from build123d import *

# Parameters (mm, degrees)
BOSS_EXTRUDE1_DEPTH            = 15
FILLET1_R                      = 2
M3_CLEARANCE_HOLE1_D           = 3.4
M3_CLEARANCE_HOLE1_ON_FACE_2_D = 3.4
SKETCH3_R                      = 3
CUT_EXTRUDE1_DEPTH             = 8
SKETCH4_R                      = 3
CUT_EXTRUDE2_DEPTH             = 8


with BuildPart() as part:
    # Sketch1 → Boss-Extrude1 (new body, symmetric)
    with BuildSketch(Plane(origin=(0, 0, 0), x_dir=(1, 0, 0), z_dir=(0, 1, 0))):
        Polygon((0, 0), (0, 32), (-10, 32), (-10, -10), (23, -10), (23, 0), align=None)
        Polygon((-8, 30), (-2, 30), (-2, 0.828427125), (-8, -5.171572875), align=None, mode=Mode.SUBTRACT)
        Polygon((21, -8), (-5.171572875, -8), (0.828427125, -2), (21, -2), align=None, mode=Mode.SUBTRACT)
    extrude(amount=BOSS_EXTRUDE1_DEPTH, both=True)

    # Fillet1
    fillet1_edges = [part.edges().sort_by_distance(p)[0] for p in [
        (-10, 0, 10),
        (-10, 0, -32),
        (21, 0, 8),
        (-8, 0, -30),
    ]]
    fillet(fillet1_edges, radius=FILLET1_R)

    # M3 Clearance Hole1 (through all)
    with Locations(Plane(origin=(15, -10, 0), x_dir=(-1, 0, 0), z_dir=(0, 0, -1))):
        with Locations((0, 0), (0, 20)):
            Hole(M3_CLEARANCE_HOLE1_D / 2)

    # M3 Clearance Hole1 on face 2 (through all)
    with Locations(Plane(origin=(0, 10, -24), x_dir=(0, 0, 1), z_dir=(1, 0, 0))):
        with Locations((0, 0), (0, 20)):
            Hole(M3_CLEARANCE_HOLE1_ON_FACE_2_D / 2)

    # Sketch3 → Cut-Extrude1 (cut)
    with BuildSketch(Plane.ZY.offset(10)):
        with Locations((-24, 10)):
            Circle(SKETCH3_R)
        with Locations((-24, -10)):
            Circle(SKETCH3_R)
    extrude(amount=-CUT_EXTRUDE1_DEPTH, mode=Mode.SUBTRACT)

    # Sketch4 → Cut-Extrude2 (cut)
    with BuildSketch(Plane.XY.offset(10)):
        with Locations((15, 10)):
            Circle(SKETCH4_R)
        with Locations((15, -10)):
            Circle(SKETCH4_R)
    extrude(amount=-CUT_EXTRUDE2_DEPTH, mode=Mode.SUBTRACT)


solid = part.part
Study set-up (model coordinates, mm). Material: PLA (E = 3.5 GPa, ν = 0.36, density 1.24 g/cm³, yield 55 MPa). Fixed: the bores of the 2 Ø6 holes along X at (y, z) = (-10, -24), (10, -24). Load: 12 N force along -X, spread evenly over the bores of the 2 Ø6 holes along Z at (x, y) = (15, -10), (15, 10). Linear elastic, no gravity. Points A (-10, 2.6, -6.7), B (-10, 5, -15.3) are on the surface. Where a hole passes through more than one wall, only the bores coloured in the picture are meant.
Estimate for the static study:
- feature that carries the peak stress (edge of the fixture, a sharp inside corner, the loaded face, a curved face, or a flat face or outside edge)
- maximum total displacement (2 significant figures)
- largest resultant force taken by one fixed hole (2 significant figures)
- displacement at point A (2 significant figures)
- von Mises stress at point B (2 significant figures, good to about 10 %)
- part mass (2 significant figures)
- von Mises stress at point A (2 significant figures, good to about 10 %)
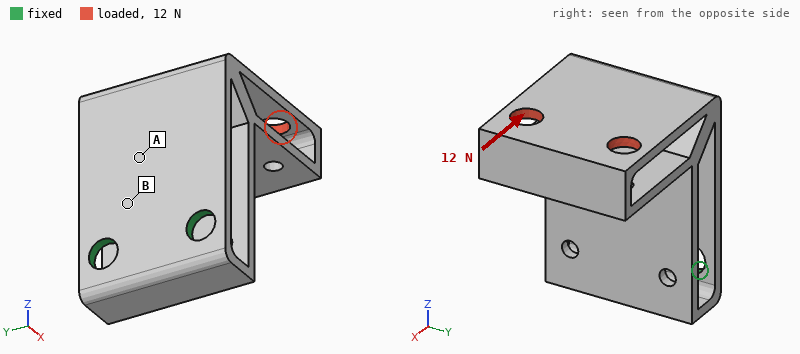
a flat face or outside edge
0.67 mm
6.4 N
0.23 mm
5.5 MPa
11 g
1.5 MPa
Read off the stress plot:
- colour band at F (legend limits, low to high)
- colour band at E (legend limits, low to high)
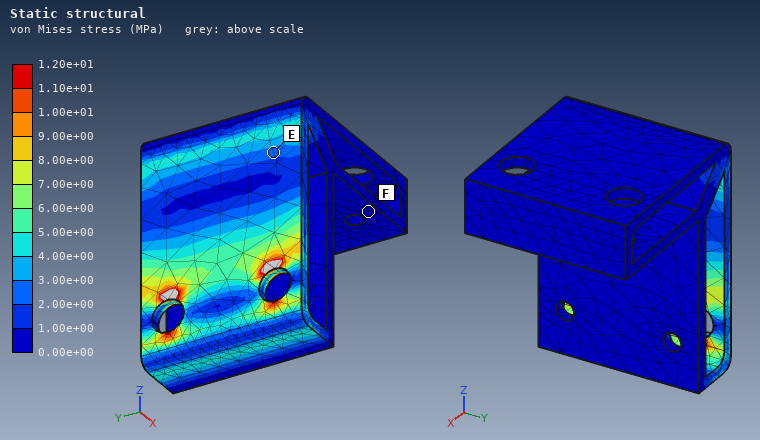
0.00e+00 to 1.00e+00 MPa
2.00e+00 to 3.00e+00 MPa
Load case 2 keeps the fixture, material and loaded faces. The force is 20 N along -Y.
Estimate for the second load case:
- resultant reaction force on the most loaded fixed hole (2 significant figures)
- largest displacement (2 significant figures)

42 N
0.64 mm
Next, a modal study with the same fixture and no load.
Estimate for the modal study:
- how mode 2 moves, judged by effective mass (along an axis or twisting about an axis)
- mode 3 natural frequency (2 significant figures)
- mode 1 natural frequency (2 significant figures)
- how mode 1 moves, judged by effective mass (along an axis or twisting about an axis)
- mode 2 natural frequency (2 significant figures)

along Y
730 Hz
280 Hz
along X
510 Hz
